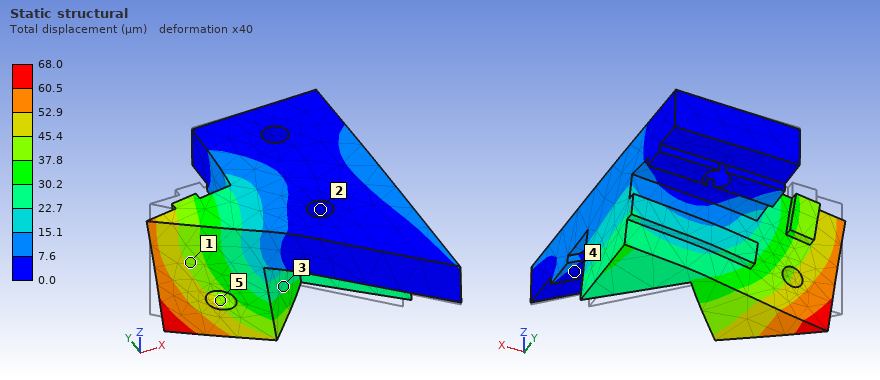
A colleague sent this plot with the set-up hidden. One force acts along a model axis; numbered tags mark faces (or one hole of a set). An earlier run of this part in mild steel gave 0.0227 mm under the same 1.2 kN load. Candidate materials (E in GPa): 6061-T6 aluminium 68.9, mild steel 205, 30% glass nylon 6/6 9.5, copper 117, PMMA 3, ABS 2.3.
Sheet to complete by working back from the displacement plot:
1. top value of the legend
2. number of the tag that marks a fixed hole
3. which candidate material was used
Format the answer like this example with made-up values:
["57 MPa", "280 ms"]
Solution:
["68.0 µm", "2", "6061-T6 aluminium"]
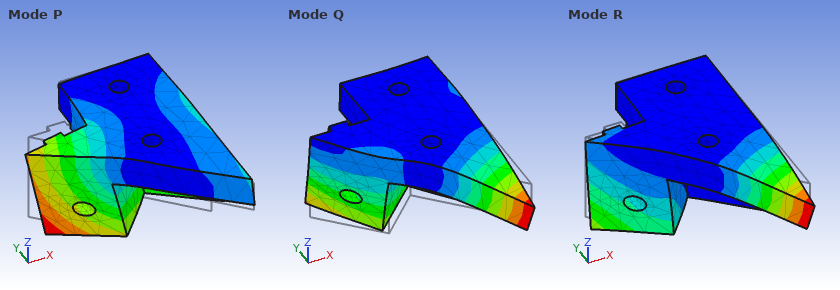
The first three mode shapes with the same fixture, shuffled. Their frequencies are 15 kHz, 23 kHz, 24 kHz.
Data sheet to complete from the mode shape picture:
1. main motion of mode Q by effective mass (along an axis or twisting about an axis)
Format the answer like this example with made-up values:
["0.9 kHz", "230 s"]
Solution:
["along Y"]
